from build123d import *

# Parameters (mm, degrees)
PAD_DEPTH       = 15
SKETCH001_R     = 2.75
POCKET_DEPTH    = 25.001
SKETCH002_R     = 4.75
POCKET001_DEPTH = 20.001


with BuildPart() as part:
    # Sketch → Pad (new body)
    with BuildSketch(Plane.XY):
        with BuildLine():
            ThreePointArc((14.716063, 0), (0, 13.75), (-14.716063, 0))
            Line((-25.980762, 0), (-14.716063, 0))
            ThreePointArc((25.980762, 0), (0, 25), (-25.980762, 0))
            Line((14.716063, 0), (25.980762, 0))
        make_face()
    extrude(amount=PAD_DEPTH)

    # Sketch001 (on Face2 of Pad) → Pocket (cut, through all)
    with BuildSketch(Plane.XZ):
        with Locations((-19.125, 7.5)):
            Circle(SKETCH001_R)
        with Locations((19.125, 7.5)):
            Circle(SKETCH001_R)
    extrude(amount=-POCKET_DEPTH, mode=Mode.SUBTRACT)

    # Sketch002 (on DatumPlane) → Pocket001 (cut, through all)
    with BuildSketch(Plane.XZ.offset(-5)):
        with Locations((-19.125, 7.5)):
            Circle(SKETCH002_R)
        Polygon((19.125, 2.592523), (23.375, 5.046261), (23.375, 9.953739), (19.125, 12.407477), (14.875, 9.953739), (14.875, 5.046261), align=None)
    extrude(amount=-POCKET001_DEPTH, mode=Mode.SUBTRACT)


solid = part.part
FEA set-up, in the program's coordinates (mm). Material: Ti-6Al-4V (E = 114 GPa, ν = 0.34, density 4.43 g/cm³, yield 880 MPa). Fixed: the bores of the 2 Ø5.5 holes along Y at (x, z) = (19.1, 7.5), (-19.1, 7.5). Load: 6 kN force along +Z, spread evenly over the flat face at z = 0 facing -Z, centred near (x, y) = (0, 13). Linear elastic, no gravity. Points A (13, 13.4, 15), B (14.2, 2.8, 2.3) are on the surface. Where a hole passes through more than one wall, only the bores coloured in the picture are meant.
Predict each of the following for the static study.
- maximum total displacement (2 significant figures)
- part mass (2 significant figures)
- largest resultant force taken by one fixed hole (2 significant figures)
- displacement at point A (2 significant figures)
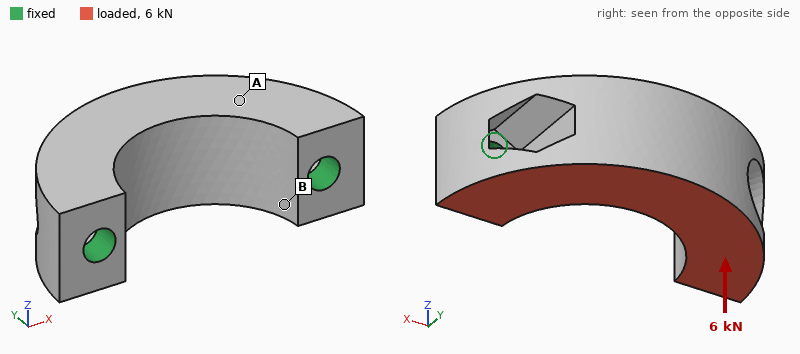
80 µm
39 g
3.0 kN
43 µm
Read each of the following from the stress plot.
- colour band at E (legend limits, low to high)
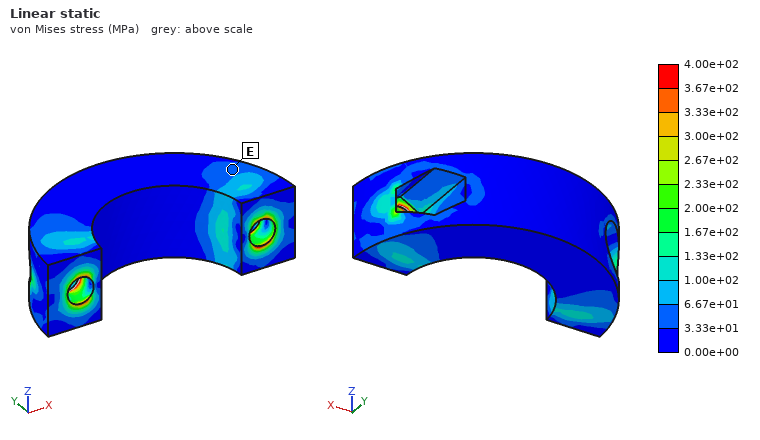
3.33e+01 to 6.67e+01 MPa
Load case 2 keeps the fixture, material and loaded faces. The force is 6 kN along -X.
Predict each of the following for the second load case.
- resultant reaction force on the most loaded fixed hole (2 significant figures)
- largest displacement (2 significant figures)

3.4 kN
26 µm
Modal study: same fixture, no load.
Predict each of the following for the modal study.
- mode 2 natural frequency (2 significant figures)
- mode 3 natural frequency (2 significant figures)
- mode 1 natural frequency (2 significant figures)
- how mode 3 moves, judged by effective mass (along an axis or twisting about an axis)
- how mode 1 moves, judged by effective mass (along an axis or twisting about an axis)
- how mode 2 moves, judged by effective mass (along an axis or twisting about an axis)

17 kHz
20 kHz
8100 Hz
twisting about Y
along Z
along X
